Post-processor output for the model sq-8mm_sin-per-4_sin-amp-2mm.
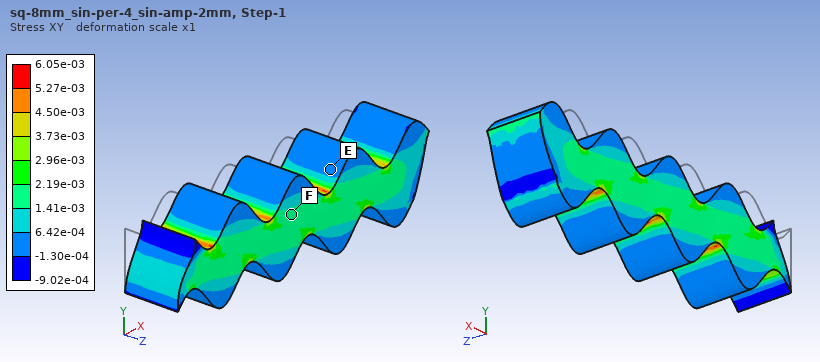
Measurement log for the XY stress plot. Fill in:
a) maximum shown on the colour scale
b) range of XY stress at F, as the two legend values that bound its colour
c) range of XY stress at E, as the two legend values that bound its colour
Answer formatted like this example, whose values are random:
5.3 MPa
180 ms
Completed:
6.05e-03
1.41e-03 to 2.19e-03
-1.30e-04 to 6.42e-04
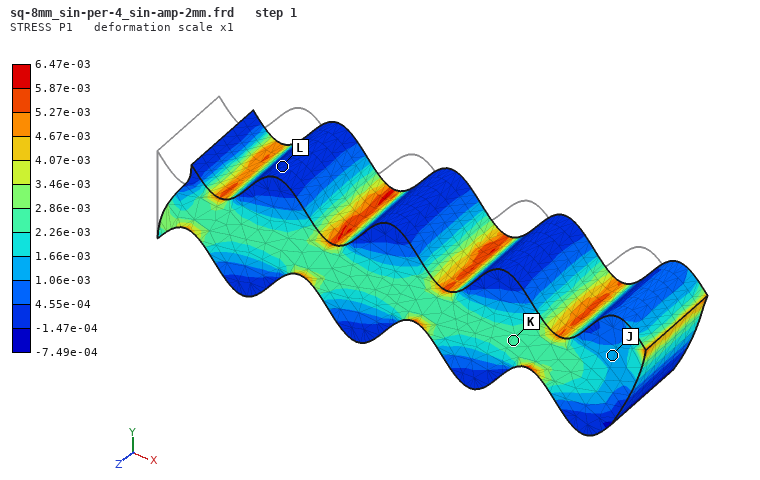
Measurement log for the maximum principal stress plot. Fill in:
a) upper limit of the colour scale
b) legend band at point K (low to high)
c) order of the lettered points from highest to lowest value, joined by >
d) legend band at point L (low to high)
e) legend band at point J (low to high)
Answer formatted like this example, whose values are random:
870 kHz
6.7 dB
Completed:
6.47e-03
2.26e-03 to 2.86e-03
K > J > L
-1.47e-04 to 4.55e-04
1.06e-03 to 1.66e-03
